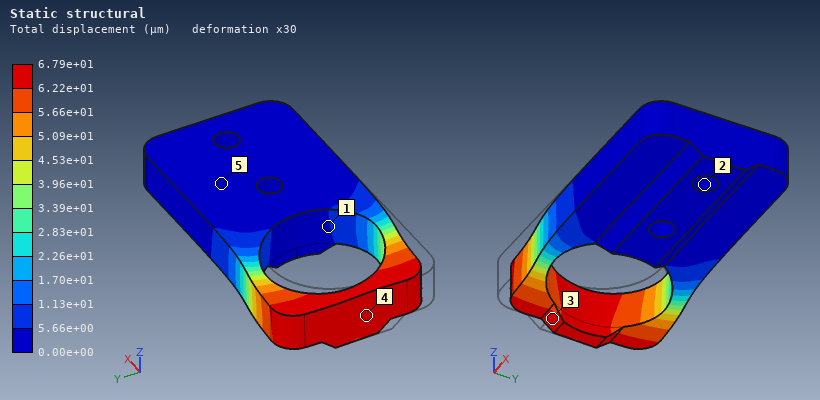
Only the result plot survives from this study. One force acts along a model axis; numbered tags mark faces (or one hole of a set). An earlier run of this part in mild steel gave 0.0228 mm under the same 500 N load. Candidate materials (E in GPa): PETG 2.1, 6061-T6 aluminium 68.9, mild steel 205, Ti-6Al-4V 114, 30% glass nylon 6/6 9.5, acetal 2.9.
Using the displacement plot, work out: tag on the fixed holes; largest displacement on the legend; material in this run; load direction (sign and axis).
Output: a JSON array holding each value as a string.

["2", "6.79e+01 µm", "6061-T6 aluminium", "+Y"]
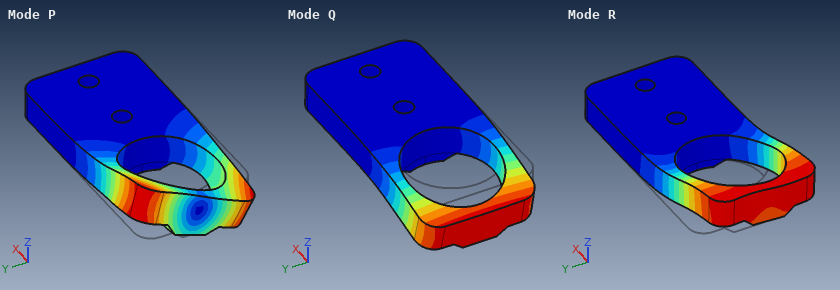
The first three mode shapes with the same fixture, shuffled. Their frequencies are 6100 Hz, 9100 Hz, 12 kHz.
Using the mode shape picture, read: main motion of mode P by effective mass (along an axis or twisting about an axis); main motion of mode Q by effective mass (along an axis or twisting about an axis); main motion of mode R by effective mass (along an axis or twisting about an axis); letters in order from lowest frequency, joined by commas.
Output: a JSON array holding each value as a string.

["twisting about X", "along Z", "along Y", "Q, R, P"]
